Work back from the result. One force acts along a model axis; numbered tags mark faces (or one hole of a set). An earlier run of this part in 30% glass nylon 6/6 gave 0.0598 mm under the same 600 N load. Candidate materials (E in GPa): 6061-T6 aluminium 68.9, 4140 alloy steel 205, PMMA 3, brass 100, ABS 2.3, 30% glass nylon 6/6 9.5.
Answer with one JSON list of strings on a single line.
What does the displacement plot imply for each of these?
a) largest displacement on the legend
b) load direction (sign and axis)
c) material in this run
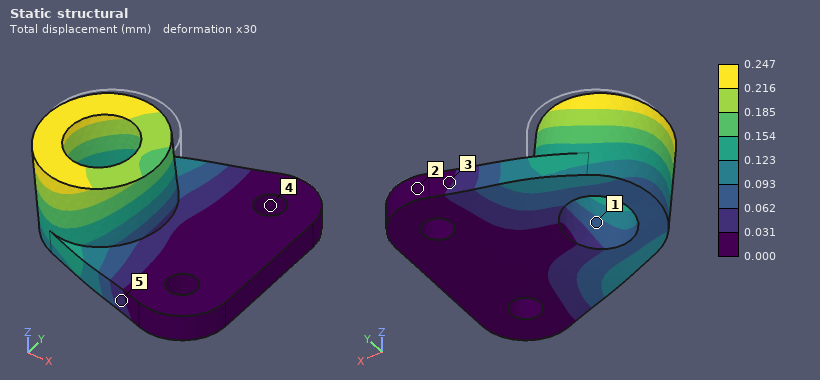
["0.247 mm", "-Y", "ABS"]
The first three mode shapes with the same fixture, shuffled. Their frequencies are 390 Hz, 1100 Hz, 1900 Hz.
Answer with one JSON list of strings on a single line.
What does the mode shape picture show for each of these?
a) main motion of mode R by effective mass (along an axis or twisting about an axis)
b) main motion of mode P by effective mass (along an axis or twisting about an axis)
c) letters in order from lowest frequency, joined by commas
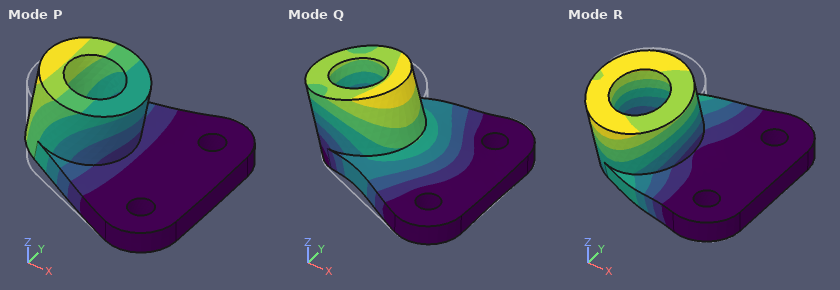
["along Y", "along Z", "P, R, Q"]
